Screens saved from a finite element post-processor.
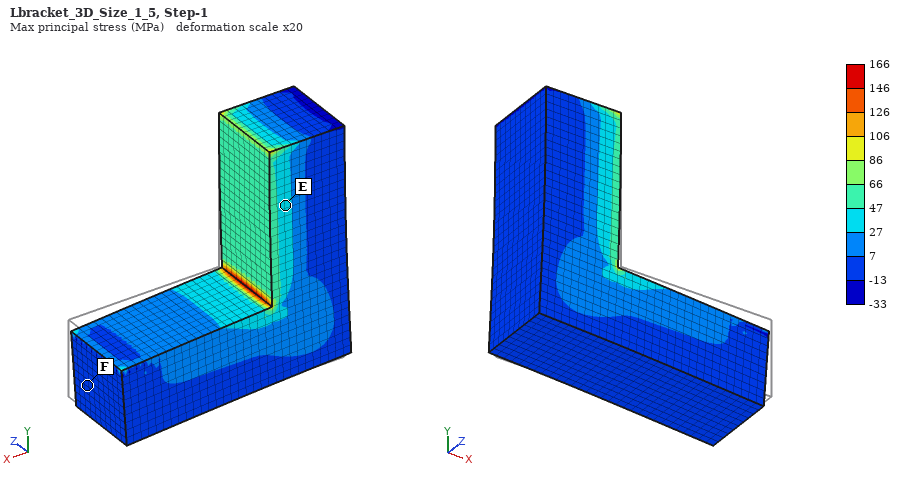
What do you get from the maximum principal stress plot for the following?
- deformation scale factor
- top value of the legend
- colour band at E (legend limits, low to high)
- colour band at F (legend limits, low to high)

20
166 MPa
27 to 47 MPa
-13 to 7 MPa
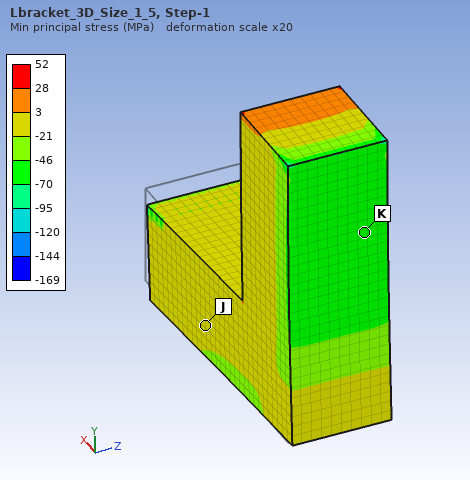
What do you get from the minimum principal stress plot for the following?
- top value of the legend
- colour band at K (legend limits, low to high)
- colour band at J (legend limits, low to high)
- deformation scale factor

52 MPa
-70 to -46 MPa
-21 to 3 MPa
20
